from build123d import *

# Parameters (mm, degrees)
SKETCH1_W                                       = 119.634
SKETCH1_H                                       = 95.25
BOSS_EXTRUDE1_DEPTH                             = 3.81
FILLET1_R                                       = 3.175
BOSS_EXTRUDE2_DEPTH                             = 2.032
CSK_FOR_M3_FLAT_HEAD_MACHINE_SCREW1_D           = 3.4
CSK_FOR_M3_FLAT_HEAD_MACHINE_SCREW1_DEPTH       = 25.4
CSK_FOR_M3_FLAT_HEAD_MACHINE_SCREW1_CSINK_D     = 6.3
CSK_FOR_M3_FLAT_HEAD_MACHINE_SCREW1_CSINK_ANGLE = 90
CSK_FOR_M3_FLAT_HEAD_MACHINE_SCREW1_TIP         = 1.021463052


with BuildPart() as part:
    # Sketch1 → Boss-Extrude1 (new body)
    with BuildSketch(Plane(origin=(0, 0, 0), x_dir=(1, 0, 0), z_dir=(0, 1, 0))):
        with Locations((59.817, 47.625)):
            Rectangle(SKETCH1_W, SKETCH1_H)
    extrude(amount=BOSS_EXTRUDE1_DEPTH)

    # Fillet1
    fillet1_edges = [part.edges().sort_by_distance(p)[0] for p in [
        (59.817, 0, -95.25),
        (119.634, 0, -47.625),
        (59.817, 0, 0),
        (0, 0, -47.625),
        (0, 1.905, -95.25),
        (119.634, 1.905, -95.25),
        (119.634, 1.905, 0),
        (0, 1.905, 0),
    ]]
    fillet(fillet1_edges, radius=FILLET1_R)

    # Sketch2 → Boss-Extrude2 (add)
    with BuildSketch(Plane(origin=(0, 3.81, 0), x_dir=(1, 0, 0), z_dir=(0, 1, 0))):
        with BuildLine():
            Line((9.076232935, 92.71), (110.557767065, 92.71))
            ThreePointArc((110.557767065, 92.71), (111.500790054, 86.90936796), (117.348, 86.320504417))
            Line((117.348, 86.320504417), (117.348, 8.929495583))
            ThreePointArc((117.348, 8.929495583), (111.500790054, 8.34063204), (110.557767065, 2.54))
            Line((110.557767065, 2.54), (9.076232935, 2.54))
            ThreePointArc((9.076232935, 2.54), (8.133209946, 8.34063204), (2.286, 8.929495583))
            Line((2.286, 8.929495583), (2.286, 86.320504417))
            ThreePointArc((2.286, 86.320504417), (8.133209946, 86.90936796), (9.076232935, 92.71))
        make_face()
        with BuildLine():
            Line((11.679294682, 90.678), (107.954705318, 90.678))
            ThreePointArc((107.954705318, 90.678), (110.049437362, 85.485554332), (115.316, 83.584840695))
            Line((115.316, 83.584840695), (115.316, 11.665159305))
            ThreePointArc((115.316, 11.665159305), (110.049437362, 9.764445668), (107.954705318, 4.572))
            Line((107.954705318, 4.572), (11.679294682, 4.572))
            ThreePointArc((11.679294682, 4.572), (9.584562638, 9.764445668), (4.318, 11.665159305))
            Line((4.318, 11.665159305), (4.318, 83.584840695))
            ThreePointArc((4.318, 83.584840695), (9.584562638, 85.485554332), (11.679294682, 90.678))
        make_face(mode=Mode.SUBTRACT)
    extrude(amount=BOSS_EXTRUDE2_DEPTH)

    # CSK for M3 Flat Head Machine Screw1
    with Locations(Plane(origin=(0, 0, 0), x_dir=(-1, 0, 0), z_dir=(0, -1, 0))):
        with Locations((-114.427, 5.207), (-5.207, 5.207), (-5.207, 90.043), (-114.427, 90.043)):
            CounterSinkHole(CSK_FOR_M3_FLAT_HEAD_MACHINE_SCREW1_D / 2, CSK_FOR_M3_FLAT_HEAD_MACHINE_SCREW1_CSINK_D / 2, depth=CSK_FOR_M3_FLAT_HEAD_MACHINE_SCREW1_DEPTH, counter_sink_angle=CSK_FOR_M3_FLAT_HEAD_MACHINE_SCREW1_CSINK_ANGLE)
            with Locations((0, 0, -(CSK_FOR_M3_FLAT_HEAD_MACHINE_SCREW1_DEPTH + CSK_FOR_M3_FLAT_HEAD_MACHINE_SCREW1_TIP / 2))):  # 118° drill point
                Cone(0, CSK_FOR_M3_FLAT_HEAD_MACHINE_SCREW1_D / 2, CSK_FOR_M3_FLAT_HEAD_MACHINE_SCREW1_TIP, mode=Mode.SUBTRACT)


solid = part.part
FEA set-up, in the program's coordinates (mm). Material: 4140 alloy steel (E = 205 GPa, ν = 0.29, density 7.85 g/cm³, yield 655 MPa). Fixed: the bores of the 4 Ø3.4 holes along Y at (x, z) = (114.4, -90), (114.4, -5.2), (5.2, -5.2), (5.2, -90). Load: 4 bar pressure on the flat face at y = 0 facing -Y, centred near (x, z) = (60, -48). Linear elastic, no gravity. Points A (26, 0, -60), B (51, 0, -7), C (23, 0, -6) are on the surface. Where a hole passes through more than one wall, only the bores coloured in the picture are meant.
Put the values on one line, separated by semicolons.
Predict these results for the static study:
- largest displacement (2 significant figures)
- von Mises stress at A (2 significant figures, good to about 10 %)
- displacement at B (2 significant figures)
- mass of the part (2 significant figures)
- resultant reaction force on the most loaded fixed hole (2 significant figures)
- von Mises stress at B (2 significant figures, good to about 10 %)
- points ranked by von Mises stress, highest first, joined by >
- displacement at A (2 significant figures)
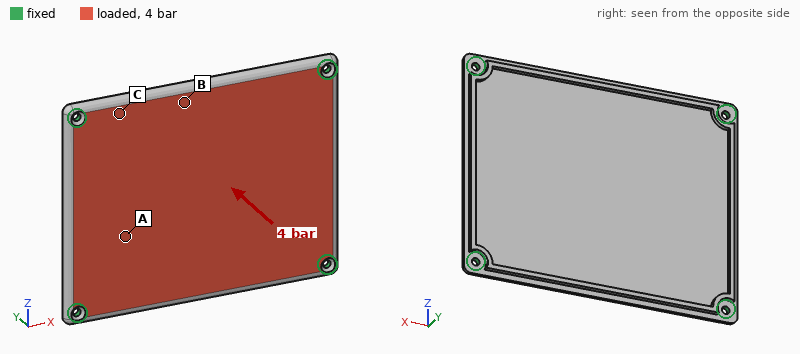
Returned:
0.34 mm; 66 MPa; 0.26 mm; 340 g; 1.4 kN; 110 MPa; B > A > C; 0.22 mm
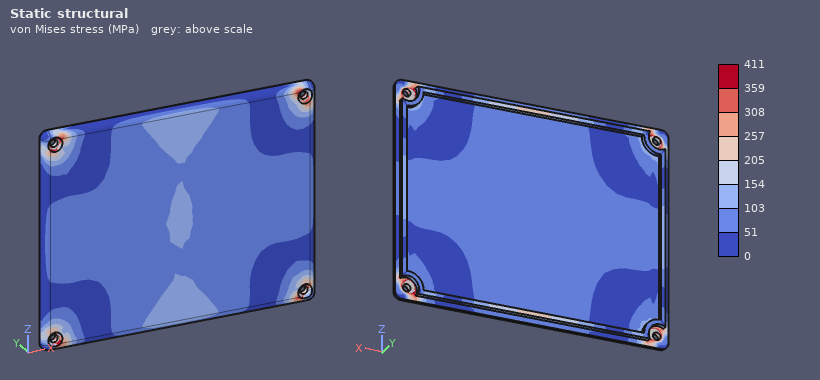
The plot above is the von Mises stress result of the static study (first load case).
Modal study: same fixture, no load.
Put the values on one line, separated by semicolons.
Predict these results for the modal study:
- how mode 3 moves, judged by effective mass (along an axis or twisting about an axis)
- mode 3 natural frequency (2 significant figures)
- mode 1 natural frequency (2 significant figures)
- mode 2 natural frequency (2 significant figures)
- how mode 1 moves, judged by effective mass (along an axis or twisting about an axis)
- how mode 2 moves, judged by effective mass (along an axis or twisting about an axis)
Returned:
twisting about Z; 2500 Hz; 1100 Hz; 2000 Hz; along Y; twisting about X
